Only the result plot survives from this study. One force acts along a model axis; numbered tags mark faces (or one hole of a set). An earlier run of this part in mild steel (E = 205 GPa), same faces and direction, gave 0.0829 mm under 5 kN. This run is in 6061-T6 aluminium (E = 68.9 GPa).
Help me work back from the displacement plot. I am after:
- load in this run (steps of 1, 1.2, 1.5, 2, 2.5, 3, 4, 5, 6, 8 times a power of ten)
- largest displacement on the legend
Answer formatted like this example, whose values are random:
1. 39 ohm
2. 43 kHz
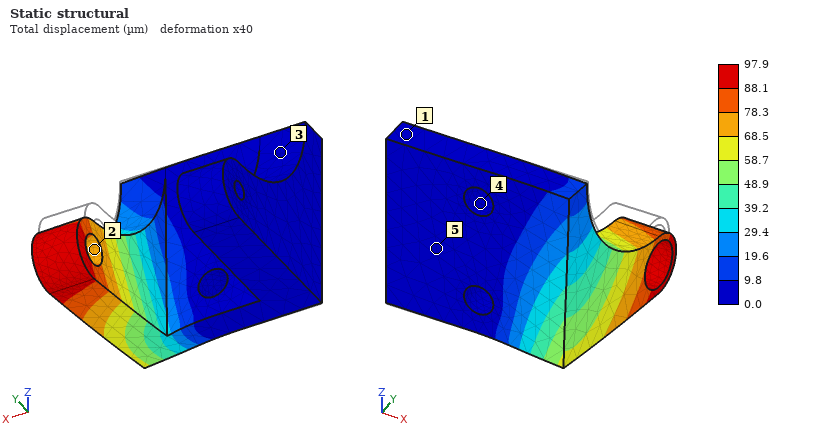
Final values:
1. 2 kN
2. 97.9 µm
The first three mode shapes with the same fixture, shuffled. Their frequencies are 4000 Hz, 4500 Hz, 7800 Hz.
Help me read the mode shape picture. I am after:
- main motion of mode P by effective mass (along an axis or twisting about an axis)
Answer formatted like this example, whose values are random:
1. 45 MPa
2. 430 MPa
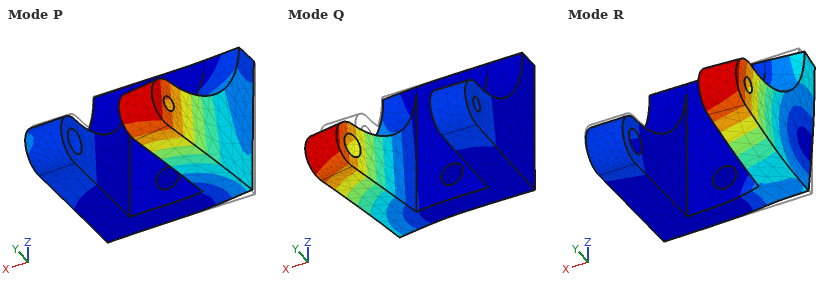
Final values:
1. along X
